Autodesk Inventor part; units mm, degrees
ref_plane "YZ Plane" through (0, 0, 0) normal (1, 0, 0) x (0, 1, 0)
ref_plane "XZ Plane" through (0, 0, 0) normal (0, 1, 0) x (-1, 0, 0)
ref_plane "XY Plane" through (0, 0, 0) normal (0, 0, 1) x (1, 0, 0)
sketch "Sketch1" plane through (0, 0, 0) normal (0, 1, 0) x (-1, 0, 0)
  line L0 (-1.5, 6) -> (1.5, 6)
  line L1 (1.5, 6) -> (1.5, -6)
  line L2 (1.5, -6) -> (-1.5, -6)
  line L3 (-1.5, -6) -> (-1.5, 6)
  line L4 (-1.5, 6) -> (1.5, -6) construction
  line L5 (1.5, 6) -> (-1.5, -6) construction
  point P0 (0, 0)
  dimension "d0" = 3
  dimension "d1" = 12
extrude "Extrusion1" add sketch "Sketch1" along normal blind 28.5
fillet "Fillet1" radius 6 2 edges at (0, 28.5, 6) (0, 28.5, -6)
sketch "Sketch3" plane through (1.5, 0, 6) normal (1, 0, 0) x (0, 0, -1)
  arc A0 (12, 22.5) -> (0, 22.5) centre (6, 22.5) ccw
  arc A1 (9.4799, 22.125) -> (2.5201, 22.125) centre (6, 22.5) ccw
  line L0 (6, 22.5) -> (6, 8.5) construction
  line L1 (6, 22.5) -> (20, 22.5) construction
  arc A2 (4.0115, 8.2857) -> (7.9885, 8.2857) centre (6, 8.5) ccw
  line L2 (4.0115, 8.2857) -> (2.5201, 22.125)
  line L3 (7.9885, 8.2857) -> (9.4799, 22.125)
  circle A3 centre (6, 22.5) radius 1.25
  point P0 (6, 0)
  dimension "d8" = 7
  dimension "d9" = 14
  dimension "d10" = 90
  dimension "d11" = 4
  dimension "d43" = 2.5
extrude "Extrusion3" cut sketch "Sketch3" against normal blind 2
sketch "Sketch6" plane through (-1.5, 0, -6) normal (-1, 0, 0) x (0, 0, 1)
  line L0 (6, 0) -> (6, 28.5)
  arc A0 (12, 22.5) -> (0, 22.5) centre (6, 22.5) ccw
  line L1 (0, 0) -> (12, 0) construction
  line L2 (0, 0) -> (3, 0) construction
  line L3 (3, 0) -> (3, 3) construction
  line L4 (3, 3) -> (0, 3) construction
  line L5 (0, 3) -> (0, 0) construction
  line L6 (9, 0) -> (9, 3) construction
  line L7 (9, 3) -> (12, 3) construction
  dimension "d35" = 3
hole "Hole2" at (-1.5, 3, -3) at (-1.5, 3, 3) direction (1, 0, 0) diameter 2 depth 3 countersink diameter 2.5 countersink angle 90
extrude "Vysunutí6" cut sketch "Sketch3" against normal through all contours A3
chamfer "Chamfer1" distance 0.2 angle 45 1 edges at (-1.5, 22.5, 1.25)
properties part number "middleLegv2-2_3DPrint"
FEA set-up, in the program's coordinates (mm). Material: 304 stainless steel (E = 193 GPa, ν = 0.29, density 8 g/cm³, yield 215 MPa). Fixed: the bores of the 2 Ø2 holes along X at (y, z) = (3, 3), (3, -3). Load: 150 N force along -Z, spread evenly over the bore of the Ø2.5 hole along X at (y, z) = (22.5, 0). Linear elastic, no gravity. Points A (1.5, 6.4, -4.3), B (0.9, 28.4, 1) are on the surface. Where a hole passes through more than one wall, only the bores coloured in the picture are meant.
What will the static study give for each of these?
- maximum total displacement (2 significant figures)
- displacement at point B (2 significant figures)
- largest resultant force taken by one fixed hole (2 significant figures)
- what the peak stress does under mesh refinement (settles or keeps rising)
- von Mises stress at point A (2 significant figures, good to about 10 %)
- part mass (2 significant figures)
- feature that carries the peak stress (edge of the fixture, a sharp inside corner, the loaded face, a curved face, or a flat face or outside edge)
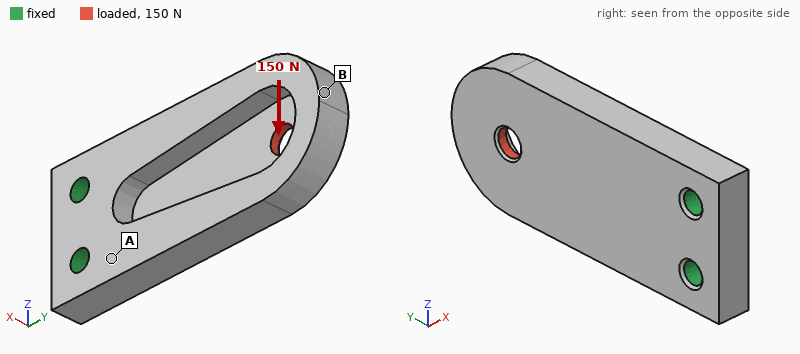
12 µm
12 µm
390 N
keeps rising
23 MPa
6.0 g
edge of the fixture
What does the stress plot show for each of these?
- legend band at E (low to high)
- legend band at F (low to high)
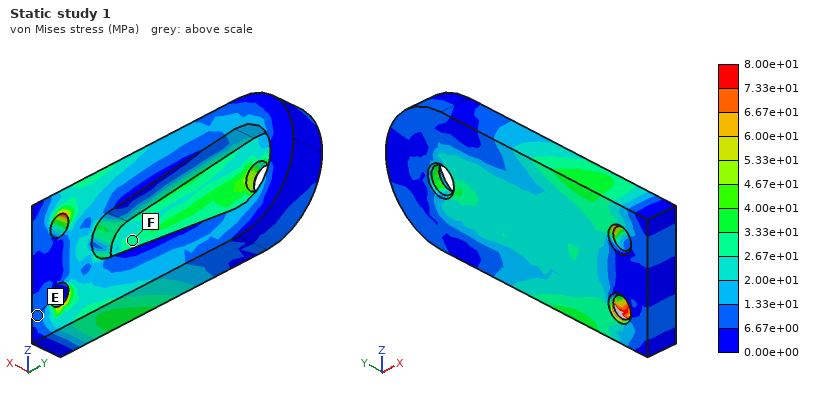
6.67e+00 to 1.33e+01 MPa
2.67e+01 to 3.33e+01 MPa
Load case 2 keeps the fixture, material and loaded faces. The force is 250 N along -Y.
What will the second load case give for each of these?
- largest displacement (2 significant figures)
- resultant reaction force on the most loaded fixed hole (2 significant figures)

13 µm
130 N
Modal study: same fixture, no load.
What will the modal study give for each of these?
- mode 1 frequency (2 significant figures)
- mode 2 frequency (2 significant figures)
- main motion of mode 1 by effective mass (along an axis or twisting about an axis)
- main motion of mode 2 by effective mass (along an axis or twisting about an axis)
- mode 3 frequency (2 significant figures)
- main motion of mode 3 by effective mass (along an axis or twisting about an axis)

4300 Hz
11 kHz
along X
along Z
15 kHz
along Z
